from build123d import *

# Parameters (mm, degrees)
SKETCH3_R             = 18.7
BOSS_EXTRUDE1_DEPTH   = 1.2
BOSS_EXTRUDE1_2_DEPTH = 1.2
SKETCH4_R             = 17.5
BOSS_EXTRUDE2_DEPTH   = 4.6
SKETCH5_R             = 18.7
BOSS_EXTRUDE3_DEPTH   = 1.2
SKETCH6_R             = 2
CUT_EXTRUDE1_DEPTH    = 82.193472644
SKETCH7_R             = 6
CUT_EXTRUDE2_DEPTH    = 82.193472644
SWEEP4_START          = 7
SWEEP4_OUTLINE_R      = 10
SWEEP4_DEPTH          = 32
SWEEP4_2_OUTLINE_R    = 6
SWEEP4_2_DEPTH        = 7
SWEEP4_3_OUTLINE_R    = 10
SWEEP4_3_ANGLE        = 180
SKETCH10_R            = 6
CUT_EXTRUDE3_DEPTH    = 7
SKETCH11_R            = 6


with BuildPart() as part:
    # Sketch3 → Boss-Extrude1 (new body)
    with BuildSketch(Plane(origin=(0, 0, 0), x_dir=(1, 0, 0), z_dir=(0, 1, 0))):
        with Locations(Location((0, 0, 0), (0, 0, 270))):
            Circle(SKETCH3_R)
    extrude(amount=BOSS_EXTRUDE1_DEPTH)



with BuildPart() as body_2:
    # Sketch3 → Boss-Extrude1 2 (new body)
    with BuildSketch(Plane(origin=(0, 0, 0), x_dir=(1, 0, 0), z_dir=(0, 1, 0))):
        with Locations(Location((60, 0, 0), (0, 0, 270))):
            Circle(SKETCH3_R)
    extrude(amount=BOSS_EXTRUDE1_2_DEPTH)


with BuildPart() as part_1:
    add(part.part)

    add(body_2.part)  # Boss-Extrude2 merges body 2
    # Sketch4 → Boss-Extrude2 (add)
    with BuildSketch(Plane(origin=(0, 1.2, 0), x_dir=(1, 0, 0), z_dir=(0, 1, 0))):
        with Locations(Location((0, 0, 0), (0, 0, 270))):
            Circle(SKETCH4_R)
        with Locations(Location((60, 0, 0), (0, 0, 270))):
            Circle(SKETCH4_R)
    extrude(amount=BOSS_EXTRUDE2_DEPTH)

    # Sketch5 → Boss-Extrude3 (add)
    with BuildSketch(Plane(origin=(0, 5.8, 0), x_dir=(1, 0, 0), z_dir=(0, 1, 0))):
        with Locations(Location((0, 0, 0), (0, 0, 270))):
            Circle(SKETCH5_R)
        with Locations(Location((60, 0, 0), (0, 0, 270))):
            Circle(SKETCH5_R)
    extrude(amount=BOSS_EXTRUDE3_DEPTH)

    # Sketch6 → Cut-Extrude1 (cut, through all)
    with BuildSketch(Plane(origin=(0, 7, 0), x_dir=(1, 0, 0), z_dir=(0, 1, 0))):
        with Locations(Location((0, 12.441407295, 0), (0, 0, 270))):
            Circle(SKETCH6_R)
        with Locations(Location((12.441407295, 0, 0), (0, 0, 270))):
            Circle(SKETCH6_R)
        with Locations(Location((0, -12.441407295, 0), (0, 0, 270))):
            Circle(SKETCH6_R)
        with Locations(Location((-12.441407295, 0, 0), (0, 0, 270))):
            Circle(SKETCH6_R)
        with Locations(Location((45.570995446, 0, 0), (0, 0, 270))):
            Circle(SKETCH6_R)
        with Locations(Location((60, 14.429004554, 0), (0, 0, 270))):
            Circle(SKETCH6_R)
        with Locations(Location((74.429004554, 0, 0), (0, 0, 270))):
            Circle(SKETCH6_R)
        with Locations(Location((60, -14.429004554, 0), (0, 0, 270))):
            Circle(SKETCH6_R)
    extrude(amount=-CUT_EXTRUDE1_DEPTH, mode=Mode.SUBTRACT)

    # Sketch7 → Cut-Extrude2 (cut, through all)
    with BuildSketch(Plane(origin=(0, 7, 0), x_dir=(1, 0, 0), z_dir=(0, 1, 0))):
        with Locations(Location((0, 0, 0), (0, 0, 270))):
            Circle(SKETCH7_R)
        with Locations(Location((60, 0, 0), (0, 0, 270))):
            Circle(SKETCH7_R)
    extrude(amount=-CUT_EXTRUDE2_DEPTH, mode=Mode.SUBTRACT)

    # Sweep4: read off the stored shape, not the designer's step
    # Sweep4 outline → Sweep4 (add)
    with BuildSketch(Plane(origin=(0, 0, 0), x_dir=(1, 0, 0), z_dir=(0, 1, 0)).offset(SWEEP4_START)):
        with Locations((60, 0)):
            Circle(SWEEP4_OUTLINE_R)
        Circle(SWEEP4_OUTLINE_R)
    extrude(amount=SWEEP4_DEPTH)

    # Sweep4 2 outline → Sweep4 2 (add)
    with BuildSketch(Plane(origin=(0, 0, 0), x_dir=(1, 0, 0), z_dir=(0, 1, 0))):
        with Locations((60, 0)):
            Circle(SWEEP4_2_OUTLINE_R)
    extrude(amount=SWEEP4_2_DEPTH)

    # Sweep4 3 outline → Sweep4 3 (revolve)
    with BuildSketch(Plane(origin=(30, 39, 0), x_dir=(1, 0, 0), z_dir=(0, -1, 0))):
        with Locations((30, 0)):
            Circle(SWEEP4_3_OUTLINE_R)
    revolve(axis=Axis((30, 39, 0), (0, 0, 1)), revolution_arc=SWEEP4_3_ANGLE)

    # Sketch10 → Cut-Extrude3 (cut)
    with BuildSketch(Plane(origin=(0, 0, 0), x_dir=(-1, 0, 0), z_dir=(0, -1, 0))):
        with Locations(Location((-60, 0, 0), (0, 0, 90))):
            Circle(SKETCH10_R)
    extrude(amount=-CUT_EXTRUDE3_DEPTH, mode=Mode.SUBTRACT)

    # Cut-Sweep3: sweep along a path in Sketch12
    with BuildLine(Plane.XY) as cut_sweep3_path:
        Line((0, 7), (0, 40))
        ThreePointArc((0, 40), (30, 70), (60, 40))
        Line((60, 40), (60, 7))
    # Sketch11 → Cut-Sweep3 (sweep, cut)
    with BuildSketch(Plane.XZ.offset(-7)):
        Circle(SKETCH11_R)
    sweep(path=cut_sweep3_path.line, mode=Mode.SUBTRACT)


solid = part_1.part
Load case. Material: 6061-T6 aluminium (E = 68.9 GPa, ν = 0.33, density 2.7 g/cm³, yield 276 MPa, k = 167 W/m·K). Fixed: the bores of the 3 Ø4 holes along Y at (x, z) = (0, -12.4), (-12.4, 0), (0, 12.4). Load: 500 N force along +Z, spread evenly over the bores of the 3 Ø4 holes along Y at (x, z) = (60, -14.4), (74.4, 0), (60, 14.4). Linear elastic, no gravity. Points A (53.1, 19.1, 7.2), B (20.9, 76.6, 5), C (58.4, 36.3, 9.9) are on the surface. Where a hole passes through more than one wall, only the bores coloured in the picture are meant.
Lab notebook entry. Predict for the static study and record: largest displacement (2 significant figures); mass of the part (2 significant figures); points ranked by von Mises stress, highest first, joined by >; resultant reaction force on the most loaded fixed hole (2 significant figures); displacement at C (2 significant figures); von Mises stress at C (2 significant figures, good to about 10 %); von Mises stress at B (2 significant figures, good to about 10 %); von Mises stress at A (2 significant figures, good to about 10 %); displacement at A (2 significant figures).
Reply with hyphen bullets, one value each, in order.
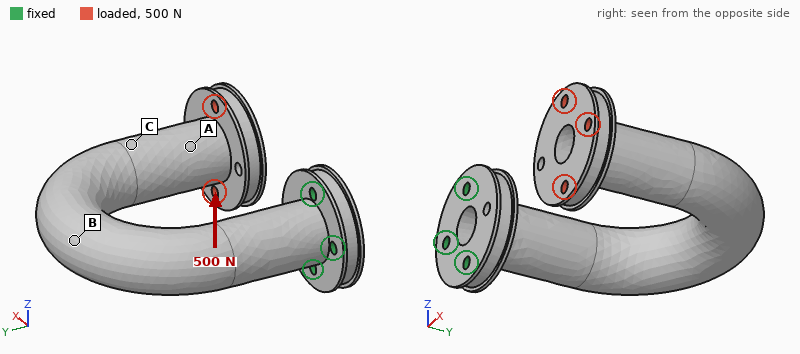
- 0.98 mm
- 120 g
- B > C > A
- 1.1 kN
- 0.54 mm
- 25 MPa
- 42 MPa
- 7.4 MPa
- 0.63 mm
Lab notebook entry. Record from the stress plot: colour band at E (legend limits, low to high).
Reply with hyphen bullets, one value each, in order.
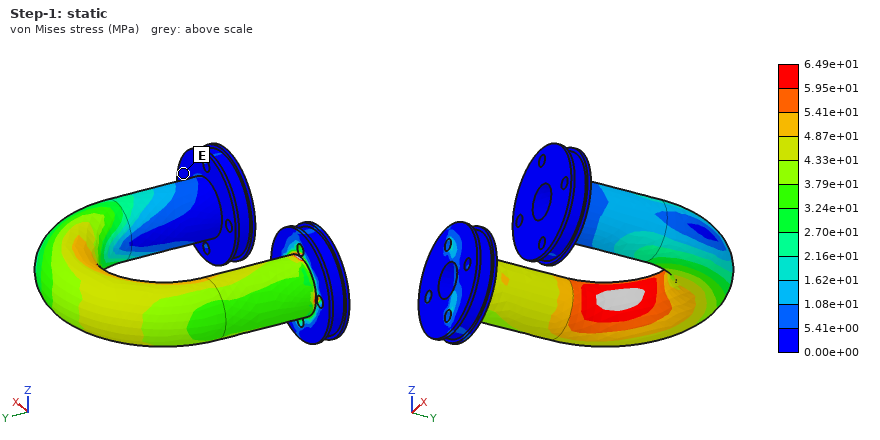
- 0.00e+00 to 5.41e+00 MPa
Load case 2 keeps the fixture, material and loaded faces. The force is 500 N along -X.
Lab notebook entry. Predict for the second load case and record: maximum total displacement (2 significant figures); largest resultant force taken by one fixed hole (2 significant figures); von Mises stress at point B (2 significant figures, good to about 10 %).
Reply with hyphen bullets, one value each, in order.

- 0.59 mm
- 190 N
- 40 MPa
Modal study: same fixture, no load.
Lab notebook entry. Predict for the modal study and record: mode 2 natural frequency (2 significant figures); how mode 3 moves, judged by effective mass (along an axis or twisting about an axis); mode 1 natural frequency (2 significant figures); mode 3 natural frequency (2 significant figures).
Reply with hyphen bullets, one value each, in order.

- 710 Hz
- along X
- 690 Hz
- 1200 Hz
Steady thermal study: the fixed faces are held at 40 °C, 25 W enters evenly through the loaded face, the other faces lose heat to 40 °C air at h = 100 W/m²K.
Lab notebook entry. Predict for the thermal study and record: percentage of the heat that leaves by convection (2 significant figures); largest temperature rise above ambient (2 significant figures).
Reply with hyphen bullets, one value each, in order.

- 92 %
- 33 K
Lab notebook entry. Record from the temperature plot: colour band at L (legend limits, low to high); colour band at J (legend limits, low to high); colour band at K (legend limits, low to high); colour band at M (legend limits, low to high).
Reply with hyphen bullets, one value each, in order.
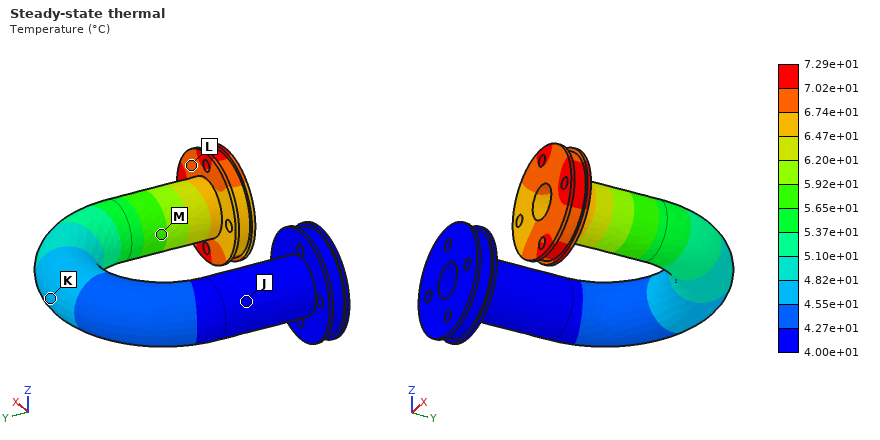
- 6.74e+01 to 7.02e+01 °C
- 4.00e+01 to 4.27e+01 °C
- 4.55e+01 to 4.82e+01 °C
- 5.65e+01 to 5.92e+01 °C
